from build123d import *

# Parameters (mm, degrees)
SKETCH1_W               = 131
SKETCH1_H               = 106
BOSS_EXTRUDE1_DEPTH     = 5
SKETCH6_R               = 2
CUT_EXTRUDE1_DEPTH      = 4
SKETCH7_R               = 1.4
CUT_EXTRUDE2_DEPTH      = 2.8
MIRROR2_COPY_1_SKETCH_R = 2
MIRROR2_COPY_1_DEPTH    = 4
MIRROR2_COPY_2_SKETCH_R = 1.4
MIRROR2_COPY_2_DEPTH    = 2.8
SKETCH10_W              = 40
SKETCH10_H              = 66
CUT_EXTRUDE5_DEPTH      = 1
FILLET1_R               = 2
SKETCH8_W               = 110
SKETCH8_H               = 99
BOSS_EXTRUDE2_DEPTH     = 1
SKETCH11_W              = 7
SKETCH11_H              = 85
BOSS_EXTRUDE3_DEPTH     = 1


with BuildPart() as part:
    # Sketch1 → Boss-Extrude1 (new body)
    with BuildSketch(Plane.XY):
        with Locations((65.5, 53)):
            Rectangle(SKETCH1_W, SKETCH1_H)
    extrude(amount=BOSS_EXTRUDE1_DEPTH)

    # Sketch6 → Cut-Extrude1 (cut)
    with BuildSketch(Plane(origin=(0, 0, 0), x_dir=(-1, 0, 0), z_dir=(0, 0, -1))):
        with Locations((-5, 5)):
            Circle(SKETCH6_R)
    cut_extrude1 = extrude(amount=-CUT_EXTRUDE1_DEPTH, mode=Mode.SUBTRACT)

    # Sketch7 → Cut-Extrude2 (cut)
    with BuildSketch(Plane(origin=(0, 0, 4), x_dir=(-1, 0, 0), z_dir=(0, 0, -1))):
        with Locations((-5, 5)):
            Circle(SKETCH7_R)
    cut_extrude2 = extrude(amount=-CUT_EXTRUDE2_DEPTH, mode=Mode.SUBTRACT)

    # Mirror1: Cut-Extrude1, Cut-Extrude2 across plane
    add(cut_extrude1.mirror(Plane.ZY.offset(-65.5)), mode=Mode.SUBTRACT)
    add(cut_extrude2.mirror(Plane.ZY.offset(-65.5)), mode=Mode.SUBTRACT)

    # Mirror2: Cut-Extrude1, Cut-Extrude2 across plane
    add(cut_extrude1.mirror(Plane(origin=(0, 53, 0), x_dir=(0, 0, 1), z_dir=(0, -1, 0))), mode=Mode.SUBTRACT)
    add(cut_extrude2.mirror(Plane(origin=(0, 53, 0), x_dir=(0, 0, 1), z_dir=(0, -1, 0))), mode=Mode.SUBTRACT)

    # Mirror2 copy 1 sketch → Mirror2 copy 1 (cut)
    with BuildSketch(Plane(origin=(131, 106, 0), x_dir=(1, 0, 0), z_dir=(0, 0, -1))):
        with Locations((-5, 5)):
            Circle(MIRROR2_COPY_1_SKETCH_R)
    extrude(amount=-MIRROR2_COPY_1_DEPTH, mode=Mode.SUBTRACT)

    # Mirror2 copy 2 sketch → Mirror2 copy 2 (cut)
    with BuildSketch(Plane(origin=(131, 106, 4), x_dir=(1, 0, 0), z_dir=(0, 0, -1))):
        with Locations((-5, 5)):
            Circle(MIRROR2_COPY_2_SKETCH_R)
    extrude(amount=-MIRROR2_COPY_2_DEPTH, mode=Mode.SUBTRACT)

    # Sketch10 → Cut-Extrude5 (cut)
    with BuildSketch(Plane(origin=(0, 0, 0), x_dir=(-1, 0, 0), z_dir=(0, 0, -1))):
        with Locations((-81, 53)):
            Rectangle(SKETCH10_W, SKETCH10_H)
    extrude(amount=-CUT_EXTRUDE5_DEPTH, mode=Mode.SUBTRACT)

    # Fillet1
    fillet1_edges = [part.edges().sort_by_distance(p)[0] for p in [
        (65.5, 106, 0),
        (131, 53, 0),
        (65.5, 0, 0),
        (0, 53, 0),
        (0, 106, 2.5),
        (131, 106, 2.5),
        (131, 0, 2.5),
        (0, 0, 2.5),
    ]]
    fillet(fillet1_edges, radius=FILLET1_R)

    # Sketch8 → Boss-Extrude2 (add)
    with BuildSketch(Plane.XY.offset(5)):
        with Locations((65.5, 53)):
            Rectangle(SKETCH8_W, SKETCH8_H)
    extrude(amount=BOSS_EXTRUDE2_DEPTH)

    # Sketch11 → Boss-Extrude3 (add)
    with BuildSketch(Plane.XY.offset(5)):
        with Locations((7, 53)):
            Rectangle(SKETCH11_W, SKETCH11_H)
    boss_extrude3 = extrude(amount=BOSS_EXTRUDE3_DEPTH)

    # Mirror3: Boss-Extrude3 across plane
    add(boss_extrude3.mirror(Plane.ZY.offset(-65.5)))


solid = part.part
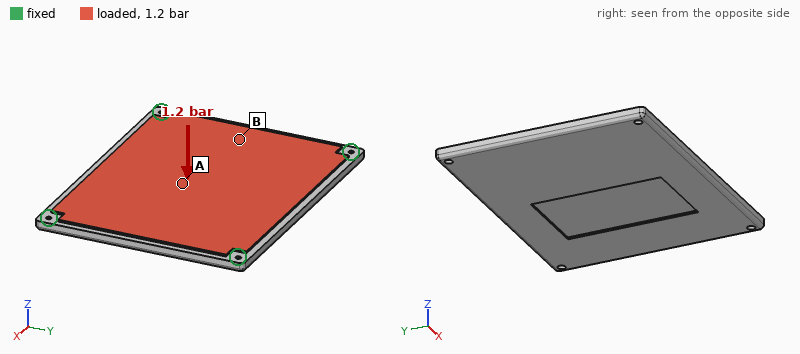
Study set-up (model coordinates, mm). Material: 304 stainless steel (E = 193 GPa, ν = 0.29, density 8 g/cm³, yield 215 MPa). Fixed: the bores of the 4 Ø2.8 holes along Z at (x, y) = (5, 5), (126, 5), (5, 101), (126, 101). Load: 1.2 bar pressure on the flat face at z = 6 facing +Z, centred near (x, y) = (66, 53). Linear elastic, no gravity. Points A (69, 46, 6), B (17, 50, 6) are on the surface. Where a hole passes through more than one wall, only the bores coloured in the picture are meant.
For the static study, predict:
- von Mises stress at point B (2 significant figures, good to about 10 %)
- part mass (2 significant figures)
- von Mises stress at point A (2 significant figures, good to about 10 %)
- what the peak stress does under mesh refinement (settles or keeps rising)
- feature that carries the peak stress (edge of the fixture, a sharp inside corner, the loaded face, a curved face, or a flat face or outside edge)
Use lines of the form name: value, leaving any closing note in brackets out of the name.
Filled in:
von Mises stress at point B: 16 MPa
part mass: 630 g
von Mises stress at point A: 27 MPa
what the peak stress does under mesh refinement: keeps rising
feature that carries the peak stress: edge of the fixture
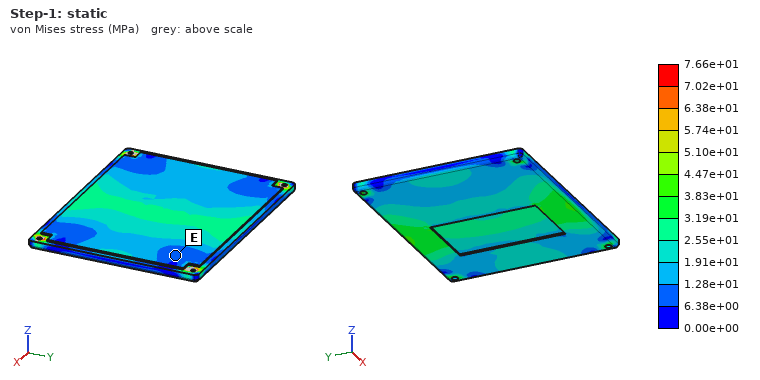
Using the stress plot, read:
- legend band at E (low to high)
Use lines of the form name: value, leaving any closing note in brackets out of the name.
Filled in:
legend band at E: 6.38e+00 to 1.28e+01 MPa
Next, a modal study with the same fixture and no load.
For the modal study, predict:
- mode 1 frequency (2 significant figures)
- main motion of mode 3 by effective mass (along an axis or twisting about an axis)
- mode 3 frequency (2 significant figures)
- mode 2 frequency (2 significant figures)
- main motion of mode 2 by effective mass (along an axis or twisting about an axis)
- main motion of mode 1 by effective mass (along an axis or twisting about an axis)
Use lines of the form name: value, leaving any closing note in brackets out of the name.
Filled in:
mode 1 frequency: 940 Hz
main motion of mode 3 by effective mass: twisting about Y
mode 3 frequency: 2200 Hz
mode 2 frequency: 1800 Hz
main motion of mode 2 by effective mass: twisting about X
main motion of mode 1 by effective mass: along Z
